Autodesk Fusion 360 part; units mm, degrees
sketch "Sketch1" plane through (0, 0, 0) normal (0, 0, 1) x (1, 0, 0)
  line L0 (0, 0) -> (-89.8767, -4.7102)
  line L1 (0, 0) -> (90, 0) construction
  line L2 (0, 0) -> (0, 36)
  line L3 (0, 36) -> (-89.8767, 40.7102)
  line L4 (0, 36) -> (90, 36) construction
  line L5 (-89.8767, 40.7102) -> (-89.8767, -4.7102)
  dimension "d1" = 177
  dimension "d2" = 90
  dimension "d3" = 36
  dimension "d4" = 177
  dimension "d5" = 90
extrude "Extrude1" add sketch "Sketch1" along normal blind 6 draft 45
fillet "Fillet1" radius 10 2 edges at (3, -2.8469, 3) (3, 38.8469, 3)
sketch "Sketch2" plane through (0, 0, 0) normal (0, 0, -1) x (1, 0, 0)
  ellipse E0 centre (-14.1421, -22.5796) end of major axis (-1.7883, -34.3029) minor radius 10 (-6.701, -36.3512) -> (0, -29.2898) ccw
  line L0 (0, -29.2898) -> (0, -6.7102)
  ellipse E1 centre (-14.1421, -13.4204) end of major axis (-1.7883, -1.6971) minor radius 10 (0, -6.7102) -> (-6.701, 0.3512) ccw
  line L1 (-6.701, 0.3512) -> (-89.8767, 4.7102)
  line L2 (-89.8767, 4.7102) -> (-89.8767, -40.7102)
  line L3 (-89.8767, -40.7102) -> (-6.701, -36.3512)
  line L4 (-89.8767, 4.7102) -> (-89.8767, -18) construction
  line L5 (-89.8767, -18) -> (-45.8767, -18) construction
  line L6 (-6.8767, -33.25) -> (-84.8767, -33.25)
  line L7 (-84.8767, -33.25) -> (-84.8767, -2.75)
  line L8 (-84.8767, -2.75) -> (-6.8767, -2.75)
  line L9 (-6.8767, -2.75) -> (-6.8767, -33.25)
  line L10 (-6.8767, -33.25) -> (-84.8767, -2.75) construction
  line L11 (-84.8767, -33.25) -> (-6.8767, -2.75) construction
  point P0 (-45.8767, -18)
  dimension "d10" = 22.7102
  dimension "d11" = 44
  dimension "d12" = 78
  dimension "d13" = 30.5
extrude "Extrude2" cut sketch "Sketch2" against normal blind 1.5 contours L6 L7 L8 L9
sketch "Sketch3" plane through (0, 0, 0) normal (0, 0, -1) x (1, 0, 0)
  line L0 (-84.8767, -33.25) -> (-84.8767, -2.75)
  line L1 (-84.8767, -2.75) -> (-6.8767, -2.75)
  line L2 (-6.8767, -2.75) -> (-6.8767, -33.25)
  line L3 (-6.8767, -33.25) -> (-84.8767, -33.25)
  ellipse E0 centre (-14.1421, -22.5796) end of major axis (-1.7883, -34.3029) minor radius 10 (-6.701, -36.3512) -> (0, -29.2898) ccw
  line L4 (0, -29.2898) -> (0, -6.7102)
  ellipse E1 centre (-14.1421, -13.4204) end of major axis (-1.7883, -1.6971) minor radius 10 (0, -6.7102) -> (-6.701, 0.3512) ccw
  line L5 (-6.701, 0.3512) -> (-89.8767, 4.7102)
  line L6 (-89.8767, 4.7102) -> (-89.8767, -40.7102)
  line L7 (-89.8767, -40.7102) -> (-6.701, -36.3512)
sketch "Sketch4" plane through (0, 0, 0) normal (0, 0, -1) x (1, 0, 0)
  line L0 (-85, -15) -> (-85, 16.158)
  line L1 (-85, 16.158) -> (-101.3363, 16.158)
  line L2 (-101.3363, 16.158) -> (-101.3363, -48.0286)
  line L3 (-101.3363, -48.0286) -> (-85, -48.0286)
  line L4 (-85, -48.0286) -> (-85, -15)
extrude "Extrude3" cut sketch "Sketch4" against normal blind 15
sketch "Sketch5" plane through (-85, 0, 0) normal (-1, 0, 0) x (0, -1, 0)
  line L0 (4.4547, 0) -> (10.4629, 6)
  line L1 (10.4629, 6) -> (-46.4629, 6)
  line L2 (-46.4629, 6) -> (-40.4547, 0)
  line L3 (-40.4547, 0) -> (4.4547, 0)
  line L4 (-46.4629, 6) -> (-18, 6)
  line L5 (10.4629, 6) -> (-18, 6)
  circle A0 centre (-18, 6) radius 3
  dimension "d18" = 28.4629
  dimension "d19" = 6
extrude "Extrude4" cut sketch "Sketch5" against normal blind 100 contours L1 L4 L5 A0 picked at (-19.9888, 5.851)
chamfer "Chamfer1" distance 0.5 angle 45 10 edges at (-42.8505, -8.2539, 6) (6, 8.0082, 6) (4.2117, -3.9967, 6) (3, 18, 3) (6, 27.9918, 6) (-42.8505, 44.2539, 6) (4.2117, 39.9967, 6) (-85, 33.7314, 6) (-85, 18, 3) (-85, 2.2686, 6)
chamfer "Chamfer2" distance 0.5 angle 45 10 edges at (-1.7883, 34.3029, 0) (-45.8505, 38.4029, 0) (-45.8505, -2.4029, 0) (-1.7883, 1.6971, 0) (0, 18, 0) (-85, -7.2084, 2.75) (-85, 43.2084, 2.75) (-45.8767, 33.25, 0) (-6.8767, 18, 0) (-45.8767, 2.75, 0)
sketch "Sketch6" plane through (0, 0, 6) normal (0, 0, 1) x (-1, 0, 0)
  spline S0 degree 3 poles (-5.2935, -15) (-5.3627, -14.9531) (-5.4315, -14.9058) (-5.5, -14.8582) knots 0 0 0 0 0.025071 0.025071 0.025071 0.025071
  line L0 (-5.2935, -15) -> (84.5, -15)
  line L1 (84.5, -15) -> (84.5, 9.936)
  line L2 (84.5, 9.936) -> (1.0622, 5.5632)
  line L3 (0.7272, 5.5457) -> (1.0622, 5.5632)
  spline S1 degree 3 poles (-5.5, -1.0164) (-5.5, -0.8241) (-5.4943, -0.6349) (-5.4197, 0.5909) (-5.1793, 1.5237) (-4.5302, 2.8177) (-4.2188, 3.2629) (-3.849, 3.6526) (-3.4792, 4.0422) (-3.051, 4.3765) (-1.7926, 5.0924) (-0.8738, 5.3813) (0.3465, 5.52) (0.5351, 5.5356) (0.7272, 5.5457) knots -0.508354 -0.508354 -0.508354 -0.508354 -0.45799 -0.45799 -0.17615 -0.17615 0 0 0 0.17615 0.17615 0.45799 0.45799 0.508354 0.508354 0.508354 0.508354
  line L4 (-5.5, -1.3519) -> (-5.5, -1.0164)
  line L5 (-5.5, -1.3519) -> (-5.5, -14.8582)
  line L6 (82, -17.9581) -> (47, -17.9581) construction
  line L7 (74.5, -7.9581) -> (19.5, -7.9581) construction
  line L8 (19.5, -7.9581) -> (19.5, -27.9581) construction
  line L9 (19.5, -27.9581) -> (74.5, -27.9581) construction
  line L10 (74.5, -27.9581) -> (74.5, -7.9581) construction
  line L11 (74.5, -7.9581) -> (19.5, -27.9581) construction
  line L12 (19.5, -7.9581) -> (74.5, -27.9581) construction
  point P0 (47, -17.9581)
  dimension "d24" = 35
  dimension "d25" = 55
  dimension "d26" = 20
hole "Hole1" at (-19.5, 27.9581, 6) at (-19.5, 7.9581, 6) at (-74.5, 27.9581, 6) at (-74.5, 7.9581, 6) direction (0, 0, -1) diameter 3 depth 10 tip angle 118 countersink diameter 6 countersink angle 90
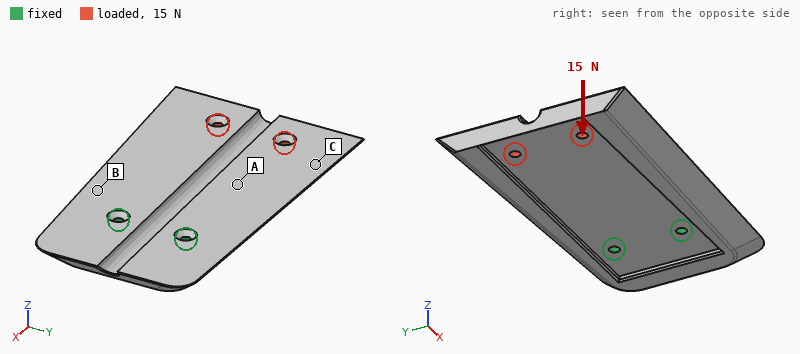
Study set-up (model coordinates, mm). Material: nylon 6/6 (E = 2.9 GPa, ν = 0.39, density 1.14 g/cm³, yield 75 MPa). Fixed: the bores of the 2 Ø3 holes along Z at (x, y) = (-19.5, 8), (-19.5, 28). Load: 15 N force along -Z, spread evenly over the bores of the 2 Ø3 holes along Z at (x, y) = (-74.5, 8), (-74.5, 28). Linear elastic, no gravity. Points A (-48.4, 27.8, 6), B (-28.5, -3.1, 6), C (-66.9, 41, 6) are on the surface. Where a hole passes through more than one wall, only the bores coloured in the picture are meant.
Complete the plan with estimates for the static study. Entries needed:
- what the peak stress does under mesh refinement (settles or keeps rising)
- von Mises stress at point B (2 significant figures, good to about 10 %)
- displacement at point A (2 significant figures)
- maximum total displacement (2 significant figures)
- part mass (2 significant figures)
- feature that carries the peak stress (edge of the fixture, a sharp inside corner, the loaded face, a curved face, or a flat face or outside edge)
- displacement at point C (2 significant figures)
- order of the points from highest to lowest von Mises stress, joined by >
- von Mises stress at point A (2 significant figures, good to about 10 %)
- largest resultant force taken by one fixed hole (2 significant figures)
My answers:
keeps rising
3.4 MPa
0.35 mm
1.1 mm
22 g
edge of the fixture
0.70 mm
B > A > C
1.9 MPa
12 N
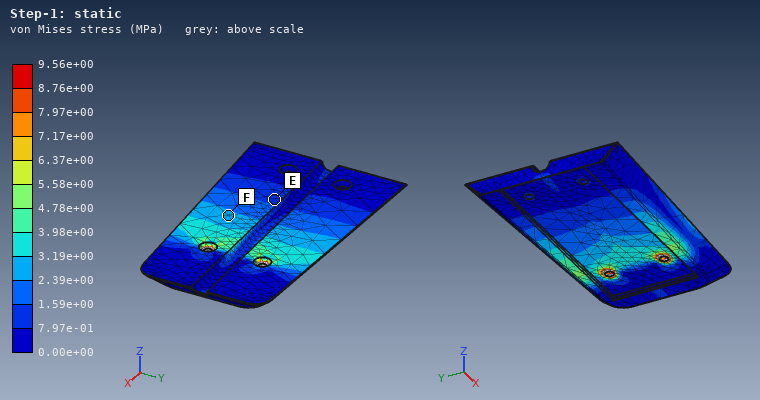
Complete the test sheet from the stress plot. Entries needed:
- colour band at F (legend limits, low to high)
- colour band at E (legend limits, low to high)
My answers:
2.39e+00 to 3.19e+00 MPa
7.97e-01 to 1.59e+00 MPa
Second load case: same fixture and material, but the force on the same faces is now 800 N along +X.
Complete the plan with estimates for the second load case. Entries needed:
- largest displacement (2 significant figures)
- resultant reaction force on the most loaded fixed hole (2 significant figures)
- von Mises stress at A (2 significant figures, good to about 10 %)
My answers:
0.73 mm
400 N
2.1 MPa
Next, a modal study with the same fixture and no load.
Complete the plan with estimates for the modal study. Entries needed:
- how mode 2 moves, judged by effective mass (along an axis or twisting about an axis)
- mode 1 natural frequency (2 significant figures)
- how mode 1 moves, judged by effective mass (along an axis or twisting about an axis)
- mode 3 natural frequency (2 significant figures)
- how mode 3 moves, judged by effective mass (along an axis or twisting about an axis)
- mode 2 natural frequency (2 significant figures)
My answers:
twisting about X
240 Hz
along Z
1300 Hz
along Y
640 Hz
